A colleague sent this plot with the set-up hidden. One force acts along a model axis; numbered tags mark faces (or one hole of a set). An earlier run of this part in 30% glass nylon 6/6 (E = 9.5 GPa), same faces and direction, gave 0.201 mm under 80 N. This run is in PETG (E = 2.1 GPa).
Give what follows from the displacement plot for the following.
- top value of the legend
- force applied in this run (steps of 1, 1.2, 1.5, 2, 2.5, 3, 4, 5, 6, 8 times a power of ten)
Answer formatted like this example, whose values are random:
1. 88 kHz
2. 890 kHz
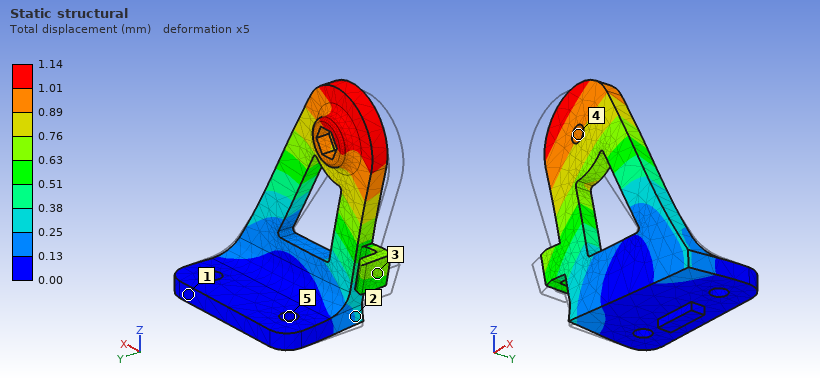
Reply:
1. 1.14 mm
2. 100 N
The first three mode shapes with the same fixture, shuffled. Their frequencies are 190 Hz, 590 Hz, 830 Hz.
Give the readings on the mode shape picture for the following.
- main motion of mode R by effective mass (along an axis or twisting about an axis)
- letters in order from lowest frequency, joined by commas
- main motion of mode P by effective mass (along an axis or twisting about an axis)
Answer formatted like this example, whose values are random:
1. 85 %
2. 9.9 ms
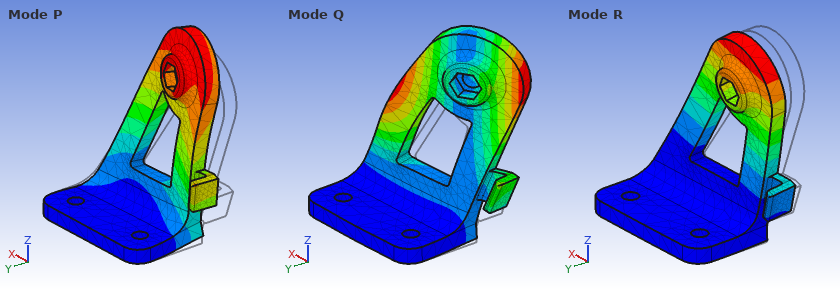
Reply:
1. along Y
2. R, P, Q
3. along X
